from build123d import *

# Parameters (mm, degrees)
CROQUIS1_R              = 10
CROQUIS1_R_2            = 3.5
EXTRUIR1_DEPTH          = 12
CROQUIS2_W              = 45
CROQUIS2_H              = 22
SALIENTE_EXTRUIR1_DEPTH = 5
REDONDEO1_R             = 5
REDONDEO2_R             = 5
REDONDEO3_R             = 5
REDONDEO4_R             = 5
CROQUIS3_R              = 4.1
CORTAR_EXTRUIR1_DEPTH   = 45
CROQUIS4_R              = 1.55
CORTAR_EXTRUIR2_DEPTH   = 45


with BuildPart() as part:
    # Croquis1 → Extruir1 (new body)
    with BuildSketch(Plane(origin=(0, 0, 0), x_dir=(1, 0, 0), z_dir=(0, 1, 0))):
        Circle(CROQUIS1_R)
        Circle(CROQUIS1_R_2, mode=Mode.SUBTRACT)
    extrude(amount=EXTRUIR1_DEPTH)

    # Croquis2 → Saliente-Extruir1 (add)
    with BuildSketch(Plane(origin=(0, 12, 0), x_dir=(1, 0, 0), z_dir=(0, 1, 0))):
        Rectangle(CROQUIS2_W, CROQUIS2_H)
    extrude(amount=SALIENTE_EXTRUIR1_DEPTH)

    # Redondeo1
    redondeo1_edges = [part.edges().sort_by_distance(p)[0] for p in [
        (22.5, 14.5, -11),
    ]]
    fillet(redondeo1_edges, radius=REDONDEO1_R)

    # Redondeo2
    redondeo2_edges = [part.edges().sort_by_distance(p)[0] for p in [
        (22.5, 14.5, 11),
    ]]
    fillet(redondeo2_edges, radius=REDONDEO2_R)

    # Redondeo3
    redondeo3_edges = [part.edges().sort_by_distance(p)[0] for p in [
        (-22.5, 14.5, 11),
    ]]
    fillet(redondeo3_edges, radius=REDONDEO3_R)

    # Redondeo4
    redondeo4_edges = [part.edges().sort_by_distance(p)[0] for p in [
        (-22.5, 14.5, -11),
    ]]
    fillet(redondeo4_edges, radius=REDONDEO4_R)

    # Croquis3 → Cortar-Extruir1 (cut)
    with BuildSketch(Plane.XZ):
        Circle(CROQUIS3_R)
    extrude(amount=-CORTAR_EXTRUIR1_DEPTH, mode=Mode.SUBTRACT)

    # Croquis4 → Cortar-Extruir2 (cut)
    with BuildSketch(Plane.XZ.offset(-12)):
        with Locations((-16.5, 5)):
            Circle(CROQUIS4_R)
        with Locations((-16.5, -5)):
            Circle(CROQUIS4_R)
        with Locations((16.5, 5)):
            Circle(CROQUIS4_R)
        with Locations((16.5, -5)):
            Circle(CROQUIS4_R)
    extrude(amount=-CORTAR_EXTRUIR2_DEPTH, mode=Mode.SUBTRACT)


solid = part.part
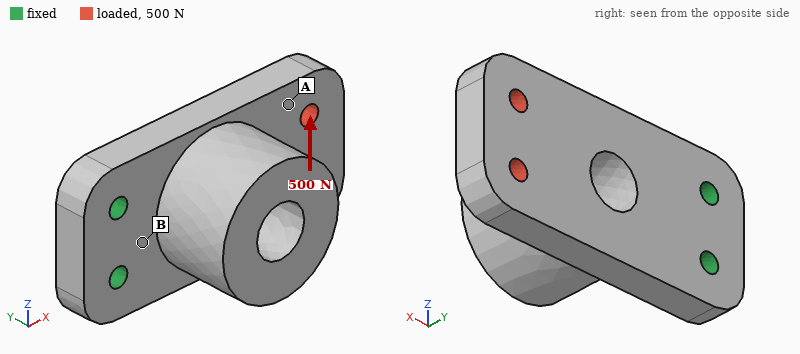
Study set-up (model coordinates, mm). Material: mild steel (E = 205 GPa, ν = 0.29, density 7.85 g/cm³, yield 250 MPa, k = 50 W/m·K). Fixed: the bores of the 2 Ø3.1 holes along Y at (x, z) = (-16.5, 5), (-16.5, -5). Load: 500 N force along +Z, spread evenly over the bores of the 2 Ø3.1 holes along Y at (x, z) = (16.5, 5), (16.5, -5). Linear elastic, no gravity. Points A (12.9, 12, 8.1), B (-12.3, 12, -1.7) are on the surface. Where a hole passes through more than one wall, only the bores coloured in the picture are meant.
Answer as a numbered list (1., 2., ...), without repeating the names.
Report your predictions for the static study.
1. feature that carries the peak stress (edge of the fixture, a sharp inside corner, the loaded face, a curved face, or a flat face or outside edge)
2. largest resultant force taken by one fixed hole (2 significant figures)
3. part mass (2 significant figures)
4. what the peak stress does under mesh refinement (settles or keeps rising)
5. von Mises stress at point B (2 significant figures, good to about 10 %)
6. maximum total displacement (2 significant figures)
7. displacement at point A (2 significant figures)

1. edge of the fixture
2. 1.4 kN
3. 59 g
4. keeps rising
5. 20 MPa
6. 14 µm
7. 9.9 µm
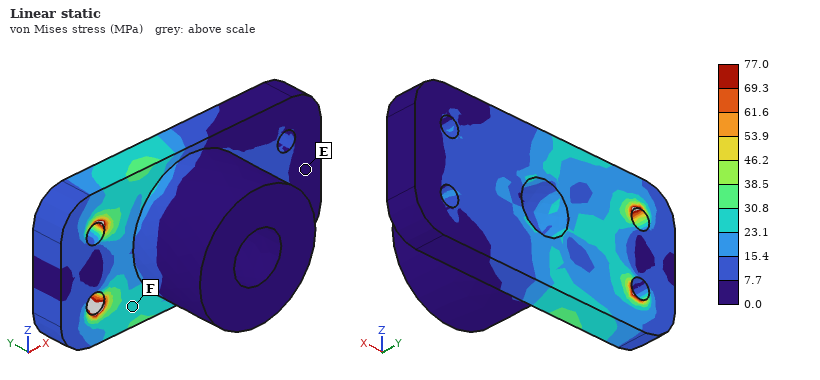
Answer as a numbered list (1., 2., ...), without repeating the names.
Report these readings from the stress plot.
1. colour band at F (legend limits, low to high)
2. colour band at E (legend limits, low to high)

1. 23.1 to 30.8 MPa
2. 0.0 to 7.7 MPa
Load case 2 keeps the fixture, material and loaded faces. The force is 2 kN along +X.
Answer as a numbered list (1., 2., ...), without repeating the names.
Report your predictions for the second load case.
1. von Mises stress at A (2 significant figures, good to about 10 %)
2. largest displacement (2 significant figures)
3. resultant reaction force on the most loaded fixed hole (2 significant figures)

1. 19 MPa
2. 7.2 µm
3. 1.0 kN
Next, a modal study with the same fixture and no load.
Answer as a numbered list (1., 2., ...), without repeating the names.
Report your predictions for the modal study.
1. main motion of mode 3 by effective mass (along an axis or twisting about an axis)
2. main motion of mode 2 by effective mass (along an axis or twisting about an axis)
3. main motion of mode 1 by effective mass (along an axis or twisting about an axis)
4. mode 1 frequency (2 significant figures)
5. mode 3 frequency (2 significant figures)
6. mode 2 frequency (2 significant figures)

1. twisting about X
2. along Z
3. along Y
4. 2600 Hz
5. 9200 Hz
6. 7300 Hz
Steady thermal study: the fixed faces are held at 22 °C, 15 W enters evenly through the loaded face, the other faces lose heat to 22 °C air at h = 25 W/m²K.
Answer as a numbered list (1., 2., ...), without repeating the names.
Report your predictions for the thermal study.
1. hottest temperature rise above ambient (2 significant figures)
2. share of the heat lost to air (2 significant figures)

1. 74 K
2. 20 %
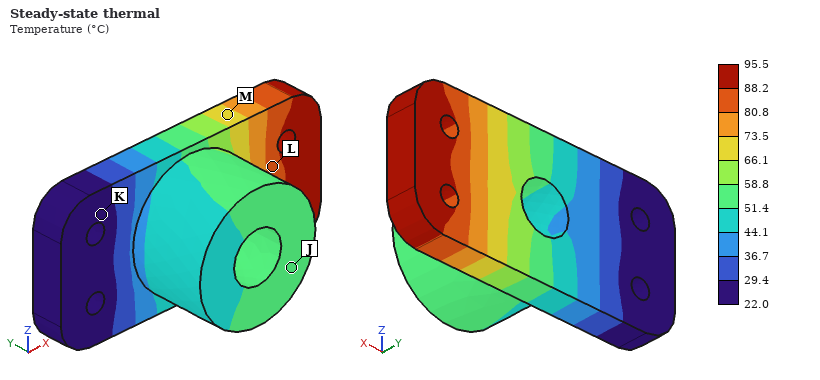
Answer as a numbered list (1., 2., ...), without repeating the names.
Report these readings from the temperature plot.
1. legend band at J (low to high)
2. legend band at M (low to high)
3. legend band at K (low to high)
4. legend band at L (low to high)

1. 51.4 to 58.8 °C
2. 66.1 to 73.5 °C
3. 22.0 to 29.4 °C
4. 80.8 to 88.2 °C
